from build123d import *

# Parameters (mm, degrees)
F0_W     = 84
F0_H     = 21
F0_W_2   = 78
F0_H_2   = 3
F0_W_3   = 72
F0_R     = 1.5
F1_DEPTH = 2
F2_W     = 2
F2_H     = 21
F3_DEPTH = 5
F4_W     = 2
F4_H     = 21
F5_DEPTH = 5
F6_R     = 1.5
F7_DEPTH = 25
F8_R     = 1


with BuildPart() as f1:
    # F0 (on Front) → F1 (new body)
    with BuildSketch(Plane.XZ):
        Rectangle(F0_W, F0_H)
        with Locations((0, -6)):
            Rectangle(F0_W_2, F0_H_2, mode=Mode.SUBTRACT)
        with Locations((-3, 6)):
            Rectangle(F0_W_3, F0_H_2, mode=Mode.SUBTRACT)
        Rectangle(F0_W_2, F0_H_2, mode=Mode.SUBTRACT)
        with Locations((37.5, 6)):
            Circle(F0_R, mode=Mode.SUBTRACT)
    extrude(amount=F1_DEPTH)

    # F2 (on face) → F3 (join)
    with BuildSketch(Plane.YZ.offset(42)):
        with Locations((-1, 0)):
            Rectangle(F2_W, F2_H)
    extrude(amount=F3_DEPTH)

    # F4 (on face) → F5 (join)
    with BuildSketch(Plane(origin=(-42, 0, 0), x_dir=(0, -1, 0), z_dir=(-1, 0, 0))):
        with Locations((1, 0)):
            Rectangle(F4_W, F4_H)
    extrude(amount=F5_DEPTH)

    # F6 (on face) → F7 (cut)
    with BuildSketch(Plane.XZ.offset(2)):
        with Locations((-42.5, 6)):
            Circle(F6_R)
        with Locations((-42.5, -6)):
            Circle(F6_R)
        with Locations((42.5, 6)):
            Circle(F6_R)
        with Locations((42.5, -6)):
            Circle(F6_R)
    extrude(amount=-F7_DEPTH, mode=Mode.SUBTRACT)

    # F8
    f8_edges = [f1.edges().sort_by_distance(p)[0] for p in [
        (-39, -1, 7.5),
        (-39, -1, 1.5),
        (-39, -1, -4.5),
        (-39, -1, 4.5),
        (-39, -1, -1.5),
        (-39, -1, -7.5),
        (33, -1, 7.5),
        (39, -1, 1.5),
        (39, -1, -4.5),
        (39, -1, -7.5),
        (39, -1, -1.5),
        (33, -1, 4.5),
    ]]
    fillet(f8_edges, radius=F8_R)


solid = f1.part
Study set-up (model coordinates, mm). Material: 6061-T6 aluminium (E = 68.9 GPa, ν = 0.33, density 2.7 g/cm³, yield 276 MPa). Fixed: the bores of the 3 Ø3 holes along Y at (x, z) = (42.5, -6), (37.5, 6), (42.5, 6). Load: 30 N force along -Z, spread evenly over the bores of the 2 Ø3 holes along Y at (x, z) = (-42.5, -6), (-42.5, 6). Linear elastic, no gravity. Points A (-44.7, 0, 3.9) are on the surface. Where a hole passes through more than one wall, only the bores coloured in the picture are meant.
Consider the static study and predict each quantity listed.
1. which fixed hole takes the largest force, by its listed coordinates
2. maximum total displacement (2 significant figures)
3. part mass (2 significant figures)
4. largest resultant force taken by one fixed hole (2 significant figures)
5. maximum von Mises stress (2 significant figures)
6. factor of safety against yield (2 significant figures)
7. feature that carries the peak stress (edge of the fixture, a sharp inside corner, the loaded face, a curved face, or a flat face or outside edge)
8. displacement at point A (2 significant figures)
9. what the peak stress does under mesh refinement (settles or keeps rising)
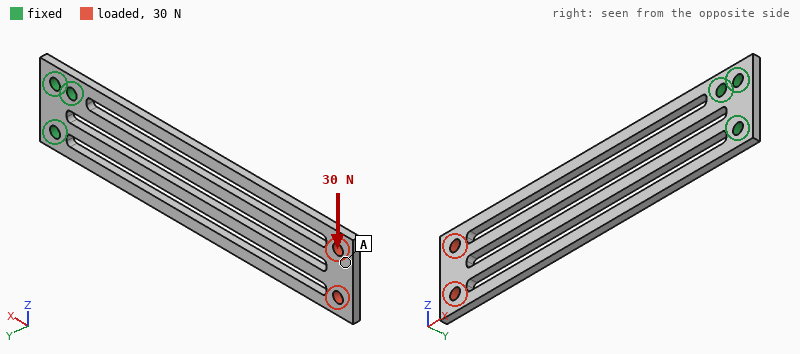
(42.5, -6)
0.99 mm
6.8 g
130 N
160 MPa
1.8
a curved face
0.98 mm
settles
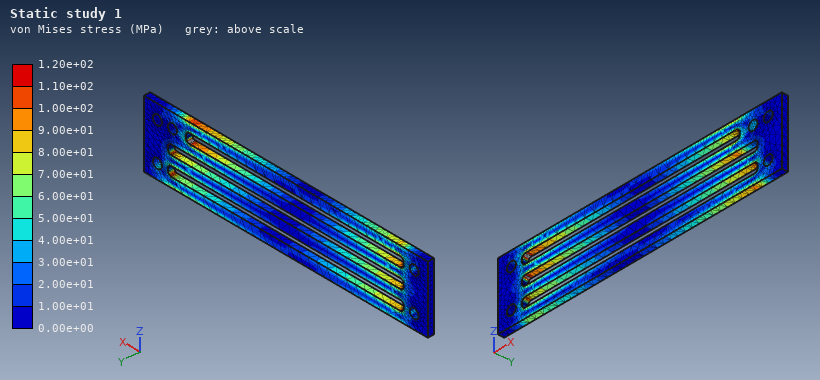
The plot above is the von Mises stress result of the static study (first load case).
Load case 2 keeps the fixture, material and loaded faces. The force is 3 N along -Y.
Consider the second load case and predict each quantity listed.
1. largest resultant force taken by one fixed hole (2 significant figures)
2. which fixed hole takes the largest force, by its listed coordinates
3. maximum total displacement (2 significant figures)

8.4 N
(37.5, 6)
1.0 mm
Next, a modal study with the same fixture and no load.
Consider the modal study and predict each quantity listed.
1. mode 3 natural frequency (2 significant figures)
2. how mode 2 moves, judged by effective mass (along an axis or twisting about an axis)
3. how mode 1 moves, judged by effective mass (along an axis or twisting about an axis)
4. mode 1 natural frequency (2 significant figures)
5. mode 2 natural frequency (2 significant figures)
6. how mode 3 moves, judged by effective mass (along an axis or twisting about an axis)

1100 Hz
along Z
along Y
210 Hz
540 Hz
twisting about X
